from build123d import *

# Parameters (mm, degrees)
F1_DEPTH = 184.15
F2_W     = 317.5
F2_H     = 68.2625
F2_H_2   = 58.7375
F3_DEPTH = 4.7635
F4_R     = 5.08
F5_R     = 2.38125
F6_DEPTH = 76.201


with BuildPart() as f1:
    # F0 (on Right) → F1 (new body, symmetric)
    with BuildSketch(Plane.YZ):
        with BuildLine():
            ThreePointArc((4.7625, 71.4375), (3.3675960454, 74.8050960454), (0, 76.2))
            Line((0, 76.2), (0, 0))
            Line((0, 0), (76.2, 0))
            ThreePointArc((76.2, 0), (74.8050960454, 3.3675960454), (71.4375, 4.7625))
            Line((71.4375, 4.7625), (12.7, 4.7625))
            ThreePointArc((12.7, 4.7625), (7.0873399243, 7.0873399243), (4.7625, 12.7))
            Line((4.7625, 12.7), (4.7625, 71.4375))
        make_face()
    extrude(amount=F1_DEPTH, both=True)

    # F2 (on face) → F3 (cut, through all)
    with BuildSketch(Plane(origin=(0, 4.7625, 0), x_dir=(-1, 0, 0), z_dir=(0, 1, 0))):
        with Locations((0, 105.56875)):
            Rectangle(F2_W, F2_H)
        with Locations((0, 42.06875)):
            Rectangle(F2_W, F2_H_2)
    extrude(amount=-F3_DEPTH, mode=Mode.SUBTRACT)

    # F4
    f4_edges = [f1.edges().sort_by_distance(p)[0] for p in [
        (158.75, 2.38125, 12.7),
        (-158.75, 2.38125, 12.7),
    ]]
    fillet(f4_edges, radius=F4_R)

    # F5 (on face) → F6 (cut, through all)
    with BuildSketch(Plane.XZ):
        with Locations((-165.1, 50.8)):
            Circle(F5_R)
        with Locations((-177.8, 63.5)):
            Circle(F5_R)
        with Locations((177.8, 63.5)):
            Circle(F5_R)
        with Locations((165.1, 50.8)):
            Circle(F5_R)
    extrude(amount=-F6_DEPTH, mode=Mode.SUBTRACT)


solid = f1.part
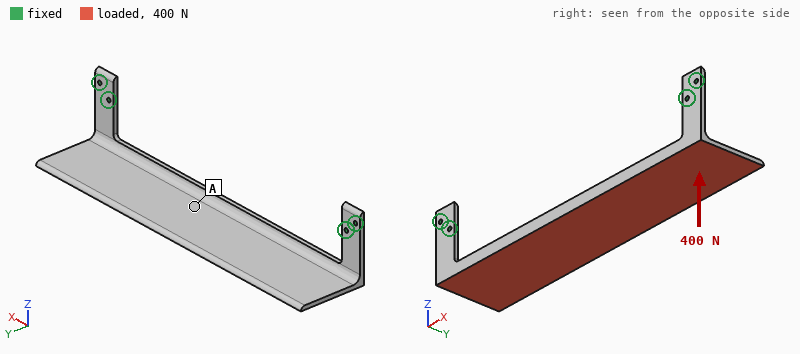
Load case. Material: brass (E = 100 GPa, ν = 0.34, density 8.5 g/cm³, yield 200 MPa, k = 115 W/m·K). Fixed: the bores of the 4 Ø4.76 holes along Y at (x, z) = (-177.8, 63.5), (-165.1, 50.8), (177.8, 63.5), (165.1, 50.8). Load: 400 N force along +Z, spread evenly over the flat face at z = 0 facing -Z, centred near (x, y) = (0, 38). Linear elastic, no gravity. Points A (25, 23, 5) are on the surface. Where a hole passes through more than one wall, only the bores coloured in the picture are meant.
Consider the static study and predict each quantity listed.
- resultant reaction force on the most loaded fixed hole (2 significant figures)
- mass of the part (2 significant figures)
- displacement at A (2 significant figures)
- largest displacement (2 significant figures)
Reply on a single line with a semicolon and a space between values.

320 N; 1.4 kg; 0.62 mm; 1.5 mm
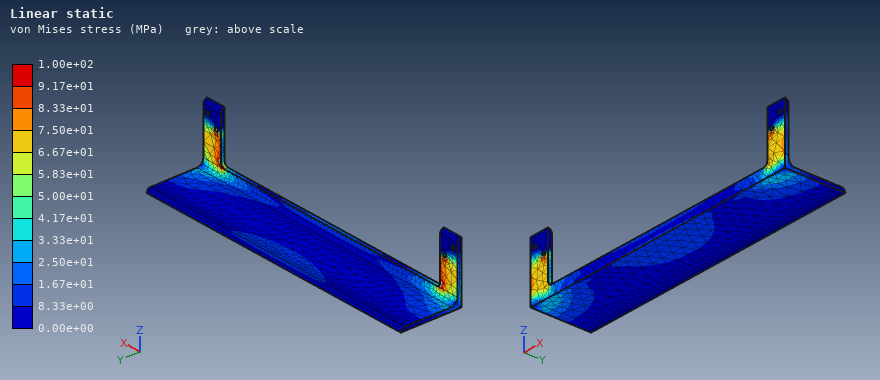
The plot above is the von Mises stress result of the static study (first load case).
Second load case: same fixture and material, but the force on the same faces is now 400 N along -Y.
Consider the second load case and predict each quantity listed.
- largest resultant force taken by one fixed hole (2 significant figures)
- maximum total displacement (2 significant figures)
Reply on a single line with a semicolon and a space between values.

440 N; 0.93 mm
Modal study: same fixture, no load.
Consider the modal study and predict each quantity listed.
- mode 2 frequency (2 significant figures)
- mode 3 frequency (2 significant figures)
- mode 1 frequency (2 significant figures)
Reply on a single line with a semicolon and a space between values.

220 Hz; 240 Hz; 90 Hz
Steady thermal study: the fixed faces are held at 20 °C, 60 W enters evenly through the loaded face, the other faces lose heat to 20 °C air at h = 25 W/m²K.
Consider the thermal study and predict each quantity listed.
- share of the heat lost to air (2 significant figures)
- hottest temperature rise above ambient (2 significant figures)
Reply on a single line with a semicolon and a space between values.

70 %; 51 K
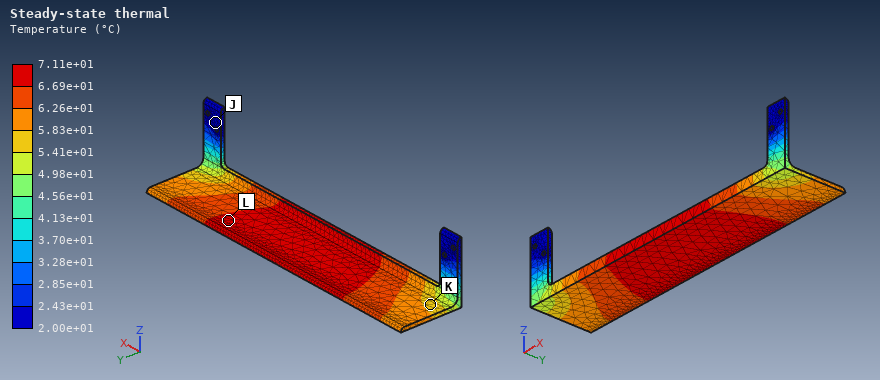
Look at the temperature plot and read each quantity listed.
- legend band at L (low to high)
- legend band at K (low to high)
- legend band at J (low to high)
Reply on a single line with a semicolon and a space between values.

6.69e+01 to 7.11e+01 °C; 5.41e+01 to 5.83e+01 °C; 2.00e+01 to 2.43e+01 °C
